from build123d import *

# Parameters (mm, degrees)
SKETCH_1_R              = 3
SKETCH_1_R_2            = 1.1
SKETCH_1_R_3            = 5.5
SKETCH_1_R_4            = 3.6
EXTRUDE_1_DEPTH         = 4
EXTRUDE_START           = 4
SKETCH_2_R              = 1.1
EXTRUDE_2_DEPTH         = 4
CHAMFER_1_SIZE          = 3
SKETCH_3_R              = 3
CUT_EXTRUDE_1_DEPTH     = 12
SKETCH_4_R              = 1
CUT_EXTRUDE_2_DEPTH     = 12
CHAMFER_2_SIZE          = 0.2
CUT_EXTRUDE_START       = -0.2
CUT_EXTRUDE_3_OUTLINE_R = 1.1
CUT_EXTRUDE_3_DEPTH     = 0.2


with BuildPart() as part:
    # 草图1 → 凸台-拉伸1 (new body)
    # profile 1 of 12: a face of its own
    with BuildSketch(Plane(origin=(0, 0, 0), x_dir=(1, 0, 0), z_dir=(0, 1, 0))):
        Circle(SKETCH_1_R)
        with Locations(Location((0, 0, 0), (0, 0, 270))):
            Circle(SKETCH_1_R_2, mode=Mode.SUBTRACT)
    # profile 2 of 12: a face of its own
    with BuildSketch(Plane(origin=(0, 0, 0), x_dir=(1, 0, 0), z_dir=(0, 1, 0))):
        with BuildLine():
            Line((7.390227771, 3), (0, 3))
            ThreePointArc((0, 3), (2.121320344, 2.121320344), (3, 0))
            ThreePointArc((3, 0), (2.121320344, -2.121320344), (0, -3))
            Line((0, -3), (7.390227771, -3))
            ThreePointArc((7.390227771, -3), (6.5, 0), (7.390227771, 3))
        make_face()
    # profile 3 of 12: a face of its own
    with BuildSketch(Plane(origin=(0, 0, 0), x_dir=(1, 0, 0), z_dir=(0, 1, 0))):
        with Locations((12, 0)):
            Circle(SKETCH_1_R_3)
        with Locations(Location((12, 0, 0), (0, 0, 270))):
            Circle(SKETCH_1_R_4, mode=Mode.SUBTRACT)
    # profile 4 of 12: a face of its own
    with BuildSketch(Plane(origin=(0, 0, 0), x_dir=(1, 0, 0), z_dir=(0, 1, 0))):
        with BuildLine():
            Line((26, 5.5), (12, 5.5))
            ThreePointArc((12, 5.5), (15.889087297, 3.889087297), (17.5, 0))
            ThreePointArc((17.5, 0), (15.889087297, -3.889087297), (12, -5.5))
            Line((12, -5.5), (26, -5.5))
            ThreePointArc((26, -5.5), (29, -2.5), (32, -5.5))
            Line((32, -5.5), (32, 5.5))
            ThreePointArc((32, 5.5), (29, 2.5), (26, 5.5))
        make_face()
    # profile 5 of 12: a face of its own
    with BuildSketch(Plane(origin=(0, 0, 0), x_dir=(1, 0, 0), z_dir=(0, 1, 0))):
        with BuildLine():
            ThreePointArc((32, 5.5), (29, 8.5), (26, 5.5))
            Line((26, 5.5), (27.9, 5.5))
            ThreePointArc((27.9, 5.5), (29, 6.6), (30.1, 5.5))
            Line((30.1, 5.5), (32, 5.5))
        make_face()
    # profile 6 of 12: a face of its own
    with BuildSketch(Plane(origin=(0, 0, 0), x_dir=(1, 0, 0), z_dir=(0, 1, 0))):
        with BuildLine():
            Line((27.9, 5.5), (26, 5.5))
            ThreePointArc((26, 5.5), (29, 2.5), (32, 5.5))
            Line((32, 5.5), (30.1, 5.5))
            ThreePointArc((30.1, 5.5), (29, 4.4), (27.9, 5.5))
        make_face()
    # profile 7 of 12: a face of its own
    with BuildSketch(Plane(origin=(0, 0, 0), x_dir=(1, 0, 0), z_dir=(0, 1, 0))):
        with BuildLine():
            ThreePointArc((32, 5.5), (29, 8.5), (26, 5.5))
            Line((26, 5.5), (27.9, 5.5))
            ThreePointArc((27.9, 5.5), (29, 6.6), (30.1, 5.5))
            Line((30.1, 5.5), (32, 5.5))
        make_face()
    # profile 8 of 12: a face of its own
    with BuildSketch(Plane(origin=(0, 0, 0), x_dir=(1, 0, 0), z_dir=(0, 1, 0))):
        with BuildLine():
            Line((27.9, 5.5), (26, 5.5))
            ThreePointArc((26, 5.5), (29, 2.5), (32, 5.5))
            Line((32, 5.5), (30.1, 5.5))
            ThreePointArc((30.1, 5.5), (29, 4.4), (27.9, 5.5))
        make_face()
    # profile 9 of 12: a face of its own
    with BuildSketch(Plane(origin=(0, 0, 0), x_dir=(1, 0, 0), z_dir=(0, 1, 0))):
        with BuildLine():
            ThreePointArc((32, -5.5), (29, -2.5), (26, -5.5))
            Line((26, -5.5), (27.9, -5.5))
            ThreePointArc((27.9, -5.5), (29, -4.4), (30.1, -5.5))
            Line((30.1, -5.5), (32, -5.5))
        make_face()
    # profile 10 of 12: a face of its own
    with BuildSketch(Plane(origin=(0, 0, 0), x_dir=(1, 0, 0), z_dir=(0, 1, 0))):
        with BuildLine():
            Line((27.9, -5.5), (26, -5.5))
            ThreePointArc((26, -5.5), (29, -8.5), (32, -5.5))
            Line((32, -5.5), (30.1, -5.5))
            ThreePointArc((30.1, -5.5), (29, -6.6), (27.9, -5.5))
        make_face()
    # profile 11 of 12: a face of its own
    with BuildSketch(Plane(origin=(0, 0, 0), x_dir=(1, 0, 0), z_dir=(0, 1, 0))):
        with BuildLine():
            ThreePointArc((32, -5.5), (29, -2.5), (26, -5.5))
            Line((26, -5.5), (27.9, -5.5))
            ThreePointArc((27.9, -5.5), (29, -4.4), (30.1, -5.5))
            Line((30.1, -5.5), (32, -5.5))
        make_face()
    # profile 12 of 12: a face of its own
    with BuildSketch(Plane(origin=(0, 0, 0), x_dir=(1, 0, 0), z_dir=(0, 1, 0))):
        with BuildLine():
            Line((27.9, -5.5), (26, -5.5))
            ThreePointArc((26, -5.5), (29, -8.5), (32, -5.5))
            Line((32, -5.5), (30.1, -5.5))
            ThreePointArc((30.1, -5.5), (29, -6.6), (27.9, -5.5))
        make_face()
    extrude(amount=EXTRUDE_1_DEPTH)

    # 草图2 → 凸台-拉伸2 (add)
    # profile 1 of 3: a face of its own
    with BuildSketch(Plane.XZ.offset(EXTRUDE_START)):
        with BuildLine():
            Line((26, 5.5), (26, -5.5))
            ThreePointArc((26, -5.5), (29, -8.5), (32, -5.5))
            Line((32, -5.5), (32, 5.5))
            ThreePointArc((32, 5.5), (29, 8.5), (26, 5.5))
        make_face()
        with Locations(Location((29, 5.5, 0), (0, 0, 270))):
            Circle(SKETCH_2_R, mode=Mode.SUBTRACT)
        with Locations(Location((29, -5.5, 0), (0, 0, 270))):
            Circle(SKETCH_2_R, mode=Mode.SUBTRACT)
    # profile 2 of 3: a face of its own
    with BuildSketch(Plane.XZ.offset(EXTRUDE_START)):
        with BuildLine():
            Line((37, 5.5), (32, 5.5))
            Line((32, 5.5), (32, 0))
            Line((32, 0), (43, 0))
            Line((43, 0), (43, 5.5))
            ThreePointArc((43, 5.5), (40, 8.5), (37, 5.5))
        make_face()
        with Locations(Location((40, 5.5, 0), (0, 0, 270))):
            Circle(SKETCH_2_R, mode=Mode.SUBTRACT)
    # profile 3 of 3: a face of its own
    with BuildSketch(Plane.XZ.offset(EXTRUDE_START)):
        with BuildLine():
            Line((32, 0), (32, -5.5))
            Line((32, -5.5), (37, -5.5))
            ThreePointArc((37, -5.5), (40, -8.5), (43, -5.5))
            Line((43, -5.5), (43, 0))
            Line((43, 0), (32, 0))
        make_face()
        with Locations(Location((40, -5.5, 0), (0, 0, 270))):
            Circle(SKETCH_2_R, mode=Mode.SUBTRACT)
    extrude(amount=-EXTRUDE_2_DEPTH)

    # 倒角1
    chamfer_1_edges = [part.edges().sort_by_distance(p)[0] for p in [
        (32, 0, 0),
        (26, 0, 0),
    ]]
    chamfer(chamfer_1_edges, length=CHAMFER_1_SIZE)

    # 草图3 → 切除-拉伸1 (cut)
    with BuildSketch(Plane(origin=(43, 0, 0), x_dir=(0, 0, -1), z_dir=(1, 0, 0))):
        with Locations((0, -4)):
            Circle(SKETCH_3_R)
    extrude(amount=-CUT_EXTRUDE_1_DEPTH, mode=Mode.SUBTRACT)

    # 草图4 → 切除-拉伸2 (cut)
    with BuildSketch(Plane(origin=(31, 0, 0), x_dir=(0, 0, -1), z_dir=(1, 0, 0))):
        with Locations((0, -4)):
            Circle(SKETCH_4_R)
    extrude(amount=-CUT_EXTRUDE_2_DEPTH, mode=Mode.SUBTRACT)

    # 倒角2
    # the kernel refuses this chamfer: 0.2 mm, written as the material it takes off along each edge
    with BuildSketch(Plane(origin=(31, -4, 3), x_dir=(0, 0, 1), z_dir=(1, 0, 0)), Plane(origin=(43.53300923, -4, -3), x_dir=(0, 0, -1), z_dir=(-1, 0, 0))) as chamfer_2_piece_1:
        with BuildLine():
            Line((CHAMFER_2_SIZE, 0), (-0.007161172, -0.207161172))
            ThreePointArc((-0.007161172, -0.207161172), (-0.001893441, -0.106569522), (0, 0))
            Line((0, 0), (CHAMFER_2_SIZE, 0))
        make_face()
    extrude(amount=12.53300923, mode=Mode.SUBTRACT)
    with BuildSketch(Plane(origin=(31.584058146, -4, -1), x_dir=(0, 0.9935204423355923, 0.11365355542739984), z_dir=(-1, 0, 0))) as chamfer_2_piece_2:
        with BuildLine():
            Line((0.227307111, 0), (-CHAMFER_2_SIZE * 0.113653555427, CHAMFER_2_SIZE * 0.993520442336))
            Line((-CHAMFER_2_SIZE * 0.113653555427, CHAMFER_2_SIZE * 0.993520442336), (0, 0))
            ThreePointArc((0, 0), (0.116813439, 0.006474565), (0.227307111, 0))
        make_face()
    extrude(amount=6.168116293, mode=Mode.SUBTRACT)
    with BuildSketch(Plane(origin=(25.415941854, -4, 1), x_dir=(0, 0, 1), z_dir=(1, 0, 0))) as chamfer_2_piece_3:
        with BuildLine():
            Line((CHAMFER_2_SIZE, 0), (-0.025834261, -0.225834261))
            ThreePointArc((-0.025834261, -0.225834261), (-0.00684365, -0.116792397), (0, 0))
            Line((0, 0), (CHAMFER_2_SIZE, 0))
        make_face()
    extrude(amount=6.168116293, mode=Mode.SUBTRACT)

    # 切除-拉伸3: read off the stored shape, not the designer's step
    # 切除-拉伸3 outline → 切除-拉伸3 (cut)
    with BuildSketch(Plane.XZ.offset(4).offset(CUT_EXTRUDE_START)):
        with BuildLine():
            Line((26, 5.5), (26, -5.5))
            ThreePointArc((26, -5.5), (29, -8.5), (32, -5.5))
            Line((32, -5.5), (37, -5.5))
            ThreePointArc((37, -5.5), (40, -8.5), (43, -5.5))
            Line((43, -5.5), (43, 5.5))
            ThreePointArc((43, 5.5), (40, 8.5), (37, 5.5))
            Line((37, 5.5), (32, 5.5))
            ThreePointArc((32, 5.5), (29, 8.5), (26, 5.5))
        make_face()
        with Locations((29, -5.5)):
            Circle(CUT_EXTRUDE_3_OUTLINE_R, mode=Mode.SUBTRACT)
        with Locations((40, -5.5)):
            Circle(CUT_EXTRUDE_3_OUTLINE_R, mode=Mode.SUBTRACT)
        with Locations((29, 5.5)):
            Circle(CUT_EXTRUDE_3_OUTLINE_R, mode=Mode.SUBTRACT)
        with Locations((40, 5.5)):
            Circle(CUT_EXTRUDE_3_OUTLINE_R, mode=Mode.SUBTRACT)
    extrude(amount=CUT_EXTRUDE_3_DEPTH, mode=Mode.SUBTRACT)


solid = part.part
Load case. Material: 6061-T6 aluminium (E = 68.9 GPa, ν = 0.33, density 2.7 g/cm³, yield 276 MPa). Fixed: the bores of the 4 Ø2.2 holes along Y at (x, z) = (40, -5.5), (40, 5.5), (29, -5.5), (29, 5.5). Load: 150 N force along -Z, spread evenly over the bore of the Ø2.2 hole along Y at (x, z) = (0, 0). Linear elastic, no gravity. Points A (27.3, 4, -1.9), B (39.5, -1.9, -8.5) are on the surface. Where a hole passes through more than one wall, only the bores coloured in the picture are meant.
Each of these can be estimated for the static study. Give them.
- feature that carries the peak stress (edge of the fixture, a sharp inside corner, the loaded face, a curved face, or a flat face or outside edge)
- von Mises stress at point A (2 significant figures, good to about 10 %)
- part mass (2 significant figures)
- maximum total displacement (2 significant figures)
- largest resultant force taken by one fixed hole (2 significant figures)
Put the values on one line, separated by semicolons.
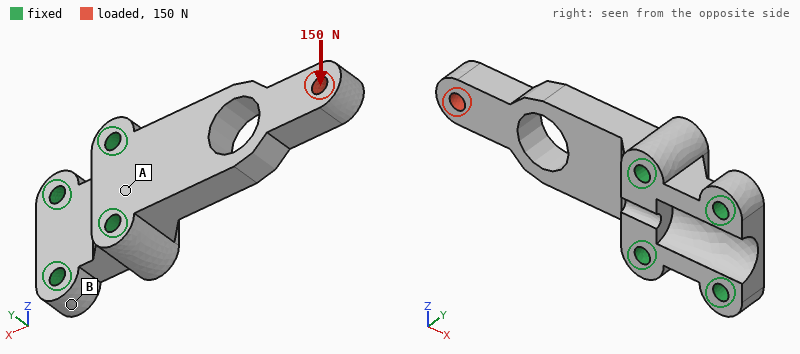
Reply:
a curved face; 11 MPa; 5.4 g; 63 µm; 400 N
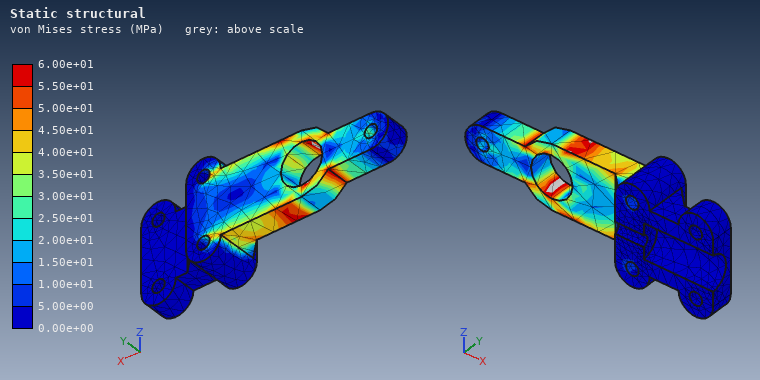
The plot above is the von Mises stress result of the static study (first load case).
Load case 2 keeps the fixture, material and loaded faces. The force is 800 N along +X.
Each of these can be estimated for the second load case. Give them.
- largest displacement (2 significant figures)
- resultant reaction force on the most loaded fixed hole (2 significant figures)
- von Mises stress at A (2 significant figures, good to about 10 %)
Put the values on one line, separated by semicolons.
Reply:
26 µm; 390 N; 13 MPa
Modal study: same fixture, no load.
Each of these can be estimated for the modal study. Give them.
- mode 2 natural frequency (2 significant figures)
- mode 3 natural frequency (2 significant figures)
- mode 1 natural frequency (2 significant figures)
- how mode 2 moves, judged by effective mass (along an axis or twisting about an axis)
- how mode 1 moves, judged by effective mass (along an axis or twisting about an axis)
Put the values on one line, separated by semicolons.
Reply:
11 kHz; 21 kHz; 4900 Hz; along Z; along Y
